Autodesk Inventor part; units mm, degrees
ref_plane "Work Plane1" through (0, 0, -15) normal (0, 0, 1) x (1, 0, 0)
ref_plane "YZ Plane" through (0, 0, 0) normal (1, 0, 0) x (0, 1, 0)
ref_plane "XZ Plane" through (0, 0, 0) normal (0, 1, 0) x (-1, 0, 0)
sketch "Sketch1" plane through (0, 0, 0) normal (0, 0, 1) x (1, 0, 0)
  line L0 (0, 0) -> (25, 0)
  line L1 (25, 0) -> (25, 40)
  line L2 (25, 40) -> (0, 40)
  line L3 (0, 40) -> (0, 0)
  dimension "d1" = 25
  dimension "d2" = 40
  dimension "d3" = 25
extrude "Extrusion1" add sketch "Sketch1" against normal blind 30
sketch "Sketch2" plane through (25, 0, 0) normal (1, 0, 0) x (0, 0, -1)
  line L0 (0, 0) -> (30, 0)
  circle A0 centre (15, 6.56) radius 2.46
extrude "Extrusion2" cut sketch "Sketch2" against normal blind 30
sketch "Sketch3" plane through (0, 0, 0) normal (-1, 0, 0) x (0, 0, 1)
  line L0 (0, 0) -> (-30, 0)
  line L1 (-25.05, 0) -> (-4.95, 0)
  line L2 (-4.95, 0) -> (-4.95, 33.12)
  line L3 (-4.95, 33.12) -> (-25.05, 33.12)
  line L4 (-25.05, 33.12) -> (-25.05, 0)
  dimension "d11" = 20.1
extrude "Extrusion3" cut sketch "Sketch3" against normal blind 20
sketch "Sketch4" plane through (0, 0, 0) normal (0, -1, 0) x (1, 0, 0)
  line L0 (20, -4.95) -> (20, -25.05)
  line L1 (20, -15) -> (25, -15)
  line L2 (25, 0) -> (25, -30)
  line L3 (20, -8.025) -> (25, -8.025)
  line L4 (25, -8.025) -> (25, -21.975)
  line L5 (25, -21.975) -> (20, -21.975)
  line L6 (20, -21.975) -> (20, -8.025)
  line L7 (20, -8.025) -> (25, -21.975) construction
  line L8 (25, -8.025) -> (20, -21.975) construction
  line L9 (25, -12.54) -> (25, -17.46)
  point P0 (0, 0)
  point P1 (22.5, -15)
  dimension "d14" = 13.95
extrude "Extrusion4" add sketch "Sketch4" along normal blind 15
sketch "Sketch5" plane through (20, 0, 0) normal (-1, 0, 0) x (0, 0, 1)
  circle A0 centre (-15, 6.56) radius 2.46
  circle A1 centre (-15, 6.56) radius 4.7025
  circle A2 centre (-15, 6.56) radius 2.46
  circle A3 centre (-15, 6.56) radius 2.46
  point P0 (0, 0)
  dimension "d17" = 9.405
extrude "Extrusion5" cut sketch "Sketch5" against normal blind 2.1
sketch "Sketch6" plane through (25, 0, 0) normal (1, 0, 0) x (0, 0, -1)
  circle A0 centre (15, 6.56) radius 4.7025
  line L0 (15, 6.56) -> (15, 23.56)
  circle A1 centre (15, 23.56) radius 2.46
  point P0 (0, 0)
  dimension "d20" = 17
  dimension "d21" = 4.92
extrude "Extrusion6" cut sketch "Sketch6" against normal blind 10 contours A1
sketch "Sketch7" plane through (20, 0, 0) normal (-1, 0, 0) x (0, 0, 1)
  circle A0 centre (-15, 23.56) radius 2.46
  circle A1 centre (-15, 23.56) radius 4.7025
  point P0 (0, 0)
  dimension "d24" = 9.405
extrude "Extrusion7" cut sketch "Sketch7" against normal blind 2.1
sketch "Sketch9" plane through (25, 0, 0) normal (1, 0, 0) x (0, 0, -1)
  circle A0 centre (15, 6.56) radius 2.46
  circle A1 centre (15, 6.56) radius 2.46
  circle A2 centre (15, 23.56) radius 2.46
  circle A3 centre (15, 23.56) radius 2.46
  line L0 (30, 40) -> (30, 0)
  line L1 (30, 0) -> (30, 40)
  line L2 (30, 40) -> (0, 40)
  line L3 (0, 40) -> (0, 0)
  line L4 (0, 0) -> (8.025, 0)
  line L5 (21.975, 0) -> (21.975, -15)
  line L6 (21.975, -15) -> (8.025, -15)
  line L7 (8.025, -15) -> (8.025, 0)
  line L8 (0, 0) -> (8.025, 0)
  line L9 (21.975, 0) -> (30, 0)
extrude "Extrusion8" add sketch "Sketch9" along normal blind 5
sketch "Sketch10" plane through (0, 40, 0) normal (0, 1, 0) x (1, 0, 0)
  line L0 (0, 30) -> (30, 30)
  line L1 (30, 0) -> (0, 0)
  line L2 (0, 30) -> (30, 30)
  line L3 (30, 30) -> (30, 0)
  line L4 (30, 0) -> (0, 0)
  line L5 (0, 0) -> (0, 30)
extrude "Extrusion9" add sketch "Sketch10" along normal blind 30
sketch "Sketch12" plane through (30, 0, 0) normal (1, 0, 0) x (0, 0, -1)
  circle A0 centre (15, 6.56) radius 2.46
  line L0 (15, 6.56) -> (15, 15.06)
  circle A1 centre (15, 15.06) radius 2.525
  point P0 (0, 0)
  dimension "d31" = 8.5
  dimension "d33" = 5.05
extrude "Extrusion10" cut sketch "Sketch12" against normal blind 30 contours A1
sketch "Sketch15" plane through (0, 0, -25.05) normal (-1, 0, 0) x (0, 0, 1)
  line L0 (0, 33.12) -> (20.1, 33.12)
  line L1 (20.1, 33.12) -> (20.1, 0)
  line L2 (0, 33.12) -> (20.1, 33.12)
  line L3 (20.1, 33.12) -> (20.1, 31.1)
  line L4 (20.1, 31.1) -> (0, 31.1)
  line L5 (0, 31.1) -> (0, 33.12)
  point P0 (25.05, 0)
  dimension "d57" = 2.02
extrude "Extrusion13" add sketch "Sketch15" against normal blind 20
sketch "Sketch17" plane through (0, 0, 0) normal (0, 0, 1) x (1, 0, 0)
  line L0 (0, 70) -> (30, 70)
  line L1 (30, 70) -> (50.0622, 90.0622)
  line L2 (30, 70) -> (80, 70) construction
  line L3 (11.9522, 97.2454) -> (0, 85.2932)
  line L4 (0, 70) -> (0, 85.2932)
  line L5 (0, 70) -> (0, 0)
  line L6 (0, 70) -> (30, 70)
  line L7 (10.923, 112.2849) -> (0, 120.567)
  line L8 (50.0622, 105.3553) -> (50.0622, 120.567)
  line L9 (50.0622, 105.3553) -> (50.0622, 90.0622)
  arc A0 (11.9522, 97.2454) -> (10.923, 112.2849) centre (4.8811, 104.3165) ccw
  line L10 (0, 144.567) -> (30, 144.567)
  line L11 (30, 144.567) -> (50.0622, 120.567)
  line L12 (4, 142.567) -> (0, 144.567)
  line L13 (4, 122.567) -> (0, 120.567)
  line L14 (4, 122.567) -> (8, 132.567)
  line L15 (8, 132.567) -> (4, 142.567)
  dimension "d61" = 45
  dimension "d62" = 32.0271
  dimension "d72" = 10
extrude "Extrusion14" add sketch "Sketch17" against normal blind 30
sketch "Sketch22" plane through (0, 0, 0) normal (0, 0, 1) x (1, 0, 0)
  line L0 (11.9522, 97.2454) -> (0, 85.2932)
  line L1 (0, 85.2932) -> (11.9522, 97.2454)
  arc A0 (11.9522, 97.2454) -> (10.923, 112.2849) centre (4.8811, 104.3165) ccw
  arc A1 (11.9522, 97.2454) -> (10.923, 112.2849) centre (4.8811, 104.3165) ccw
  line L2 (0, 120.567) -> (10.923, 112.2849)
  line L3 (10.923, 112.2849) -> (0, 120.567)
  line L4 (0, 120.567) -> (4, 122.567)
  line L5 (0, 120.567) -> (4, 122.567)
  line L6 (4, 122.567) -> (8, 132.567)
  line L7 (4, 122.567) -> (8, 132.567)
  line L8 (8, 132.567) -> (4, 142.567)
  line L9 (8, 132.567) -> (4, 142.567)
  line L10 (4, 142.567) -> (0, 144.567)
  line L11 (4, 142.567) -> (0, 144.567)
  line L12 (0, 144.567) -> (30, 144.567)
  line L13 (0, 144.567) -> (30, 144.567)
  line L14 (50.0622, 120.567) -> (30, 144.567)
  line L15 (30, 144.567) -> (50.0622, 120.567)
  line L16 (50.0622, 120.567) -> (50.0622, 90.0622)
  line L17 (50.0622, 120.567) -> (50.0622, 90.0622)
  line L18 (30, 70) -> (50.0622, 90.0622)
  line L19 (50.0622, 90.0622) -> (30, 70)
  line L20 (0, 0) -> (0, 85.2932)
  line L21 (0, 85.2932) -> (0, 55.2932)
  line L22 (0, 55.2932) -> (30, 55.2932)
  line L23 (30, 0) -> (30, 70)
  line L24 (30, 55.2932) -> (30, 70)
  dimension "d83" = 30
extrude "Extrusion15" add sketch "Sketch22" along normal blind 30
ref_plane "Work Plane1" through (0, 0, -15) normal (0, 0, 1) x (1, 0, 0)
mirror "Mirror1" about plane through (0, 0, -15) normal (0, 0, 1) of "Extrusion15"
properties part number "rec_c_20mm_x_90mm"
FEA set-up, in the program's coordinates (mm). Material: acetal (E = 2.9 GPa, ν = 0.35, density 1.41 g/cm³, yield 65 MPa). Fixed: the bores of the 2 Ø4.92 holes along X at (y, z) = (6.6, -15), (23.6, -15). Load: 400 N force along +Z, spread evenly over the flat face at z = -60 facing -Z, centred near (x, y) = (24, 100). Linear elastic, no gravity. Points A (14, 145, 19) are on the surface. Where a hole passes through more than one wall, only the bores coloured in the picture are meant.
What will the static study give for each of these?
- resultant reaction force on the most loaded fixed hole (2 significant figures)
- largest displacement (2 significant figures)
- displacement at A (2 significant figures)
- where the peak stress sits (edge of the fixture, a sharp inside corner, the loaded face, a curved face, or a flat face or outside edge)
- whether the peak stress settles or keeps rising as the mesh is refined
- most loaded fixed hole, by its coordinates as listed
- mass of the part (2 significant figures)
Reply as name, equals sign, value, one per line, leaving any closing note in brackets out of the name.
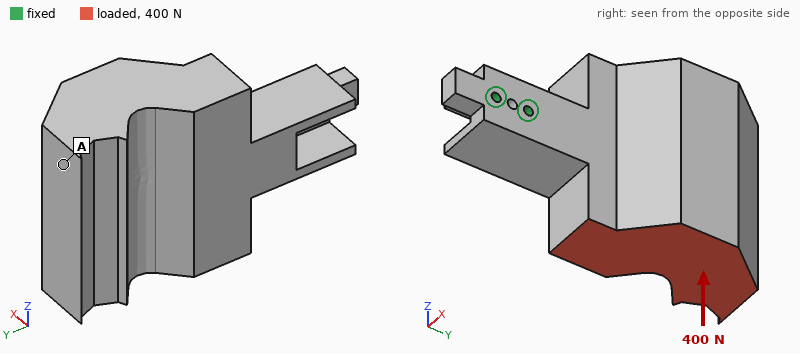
resultant reaction force on the most loaded fixed hole = 1.7 kN
largest displacement = 1.9 mm
displacement at A = 1.8 mm
where the peak stress sits = edge of the fixture
whether the peak stress settles or keeps rising as the mesh is refined = keeps rising
most loaded fixed hole, by its coordinates as listed = (23.6, -15)
mass of the part = 470 g
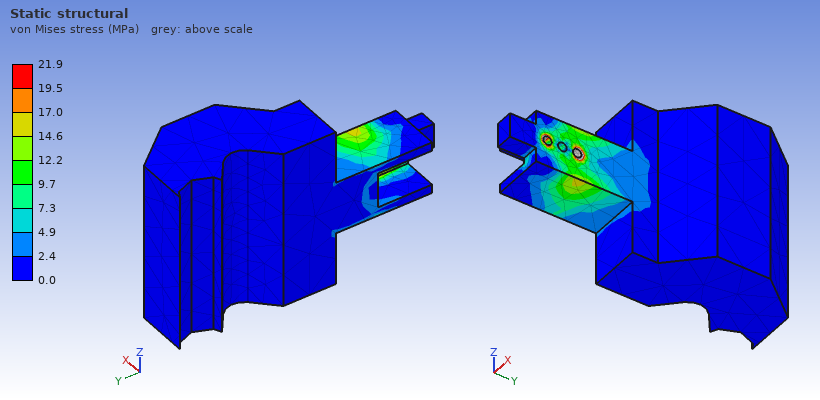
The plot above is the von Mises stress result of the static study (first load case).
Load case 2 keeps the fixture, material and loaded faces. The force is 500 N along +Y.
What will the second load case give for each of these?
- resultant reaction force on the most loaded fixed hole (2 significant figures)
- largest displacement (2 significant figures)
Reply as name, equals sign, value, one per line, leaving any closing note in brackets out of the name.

resultant reaction force on the most loaded fixed hole = 1.0 kN
largest displacement = 1.6 mm
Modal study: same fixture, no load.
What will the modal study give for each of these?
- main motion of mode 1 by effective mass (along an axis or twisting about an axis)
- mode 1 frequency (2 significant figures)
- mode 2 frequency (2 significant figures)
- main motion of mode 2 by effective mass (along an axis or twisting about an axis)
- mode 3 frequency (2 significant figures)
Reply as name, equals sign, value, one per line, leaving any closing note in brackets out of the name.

main motion of mode 1 by effective mass = along X
mode 1 frequency = 120 Hz
mode 2 frequency = 130 Hz
main motion of mode 2 by effective mass = along Z
mode 3 frequency = 230 Hz
